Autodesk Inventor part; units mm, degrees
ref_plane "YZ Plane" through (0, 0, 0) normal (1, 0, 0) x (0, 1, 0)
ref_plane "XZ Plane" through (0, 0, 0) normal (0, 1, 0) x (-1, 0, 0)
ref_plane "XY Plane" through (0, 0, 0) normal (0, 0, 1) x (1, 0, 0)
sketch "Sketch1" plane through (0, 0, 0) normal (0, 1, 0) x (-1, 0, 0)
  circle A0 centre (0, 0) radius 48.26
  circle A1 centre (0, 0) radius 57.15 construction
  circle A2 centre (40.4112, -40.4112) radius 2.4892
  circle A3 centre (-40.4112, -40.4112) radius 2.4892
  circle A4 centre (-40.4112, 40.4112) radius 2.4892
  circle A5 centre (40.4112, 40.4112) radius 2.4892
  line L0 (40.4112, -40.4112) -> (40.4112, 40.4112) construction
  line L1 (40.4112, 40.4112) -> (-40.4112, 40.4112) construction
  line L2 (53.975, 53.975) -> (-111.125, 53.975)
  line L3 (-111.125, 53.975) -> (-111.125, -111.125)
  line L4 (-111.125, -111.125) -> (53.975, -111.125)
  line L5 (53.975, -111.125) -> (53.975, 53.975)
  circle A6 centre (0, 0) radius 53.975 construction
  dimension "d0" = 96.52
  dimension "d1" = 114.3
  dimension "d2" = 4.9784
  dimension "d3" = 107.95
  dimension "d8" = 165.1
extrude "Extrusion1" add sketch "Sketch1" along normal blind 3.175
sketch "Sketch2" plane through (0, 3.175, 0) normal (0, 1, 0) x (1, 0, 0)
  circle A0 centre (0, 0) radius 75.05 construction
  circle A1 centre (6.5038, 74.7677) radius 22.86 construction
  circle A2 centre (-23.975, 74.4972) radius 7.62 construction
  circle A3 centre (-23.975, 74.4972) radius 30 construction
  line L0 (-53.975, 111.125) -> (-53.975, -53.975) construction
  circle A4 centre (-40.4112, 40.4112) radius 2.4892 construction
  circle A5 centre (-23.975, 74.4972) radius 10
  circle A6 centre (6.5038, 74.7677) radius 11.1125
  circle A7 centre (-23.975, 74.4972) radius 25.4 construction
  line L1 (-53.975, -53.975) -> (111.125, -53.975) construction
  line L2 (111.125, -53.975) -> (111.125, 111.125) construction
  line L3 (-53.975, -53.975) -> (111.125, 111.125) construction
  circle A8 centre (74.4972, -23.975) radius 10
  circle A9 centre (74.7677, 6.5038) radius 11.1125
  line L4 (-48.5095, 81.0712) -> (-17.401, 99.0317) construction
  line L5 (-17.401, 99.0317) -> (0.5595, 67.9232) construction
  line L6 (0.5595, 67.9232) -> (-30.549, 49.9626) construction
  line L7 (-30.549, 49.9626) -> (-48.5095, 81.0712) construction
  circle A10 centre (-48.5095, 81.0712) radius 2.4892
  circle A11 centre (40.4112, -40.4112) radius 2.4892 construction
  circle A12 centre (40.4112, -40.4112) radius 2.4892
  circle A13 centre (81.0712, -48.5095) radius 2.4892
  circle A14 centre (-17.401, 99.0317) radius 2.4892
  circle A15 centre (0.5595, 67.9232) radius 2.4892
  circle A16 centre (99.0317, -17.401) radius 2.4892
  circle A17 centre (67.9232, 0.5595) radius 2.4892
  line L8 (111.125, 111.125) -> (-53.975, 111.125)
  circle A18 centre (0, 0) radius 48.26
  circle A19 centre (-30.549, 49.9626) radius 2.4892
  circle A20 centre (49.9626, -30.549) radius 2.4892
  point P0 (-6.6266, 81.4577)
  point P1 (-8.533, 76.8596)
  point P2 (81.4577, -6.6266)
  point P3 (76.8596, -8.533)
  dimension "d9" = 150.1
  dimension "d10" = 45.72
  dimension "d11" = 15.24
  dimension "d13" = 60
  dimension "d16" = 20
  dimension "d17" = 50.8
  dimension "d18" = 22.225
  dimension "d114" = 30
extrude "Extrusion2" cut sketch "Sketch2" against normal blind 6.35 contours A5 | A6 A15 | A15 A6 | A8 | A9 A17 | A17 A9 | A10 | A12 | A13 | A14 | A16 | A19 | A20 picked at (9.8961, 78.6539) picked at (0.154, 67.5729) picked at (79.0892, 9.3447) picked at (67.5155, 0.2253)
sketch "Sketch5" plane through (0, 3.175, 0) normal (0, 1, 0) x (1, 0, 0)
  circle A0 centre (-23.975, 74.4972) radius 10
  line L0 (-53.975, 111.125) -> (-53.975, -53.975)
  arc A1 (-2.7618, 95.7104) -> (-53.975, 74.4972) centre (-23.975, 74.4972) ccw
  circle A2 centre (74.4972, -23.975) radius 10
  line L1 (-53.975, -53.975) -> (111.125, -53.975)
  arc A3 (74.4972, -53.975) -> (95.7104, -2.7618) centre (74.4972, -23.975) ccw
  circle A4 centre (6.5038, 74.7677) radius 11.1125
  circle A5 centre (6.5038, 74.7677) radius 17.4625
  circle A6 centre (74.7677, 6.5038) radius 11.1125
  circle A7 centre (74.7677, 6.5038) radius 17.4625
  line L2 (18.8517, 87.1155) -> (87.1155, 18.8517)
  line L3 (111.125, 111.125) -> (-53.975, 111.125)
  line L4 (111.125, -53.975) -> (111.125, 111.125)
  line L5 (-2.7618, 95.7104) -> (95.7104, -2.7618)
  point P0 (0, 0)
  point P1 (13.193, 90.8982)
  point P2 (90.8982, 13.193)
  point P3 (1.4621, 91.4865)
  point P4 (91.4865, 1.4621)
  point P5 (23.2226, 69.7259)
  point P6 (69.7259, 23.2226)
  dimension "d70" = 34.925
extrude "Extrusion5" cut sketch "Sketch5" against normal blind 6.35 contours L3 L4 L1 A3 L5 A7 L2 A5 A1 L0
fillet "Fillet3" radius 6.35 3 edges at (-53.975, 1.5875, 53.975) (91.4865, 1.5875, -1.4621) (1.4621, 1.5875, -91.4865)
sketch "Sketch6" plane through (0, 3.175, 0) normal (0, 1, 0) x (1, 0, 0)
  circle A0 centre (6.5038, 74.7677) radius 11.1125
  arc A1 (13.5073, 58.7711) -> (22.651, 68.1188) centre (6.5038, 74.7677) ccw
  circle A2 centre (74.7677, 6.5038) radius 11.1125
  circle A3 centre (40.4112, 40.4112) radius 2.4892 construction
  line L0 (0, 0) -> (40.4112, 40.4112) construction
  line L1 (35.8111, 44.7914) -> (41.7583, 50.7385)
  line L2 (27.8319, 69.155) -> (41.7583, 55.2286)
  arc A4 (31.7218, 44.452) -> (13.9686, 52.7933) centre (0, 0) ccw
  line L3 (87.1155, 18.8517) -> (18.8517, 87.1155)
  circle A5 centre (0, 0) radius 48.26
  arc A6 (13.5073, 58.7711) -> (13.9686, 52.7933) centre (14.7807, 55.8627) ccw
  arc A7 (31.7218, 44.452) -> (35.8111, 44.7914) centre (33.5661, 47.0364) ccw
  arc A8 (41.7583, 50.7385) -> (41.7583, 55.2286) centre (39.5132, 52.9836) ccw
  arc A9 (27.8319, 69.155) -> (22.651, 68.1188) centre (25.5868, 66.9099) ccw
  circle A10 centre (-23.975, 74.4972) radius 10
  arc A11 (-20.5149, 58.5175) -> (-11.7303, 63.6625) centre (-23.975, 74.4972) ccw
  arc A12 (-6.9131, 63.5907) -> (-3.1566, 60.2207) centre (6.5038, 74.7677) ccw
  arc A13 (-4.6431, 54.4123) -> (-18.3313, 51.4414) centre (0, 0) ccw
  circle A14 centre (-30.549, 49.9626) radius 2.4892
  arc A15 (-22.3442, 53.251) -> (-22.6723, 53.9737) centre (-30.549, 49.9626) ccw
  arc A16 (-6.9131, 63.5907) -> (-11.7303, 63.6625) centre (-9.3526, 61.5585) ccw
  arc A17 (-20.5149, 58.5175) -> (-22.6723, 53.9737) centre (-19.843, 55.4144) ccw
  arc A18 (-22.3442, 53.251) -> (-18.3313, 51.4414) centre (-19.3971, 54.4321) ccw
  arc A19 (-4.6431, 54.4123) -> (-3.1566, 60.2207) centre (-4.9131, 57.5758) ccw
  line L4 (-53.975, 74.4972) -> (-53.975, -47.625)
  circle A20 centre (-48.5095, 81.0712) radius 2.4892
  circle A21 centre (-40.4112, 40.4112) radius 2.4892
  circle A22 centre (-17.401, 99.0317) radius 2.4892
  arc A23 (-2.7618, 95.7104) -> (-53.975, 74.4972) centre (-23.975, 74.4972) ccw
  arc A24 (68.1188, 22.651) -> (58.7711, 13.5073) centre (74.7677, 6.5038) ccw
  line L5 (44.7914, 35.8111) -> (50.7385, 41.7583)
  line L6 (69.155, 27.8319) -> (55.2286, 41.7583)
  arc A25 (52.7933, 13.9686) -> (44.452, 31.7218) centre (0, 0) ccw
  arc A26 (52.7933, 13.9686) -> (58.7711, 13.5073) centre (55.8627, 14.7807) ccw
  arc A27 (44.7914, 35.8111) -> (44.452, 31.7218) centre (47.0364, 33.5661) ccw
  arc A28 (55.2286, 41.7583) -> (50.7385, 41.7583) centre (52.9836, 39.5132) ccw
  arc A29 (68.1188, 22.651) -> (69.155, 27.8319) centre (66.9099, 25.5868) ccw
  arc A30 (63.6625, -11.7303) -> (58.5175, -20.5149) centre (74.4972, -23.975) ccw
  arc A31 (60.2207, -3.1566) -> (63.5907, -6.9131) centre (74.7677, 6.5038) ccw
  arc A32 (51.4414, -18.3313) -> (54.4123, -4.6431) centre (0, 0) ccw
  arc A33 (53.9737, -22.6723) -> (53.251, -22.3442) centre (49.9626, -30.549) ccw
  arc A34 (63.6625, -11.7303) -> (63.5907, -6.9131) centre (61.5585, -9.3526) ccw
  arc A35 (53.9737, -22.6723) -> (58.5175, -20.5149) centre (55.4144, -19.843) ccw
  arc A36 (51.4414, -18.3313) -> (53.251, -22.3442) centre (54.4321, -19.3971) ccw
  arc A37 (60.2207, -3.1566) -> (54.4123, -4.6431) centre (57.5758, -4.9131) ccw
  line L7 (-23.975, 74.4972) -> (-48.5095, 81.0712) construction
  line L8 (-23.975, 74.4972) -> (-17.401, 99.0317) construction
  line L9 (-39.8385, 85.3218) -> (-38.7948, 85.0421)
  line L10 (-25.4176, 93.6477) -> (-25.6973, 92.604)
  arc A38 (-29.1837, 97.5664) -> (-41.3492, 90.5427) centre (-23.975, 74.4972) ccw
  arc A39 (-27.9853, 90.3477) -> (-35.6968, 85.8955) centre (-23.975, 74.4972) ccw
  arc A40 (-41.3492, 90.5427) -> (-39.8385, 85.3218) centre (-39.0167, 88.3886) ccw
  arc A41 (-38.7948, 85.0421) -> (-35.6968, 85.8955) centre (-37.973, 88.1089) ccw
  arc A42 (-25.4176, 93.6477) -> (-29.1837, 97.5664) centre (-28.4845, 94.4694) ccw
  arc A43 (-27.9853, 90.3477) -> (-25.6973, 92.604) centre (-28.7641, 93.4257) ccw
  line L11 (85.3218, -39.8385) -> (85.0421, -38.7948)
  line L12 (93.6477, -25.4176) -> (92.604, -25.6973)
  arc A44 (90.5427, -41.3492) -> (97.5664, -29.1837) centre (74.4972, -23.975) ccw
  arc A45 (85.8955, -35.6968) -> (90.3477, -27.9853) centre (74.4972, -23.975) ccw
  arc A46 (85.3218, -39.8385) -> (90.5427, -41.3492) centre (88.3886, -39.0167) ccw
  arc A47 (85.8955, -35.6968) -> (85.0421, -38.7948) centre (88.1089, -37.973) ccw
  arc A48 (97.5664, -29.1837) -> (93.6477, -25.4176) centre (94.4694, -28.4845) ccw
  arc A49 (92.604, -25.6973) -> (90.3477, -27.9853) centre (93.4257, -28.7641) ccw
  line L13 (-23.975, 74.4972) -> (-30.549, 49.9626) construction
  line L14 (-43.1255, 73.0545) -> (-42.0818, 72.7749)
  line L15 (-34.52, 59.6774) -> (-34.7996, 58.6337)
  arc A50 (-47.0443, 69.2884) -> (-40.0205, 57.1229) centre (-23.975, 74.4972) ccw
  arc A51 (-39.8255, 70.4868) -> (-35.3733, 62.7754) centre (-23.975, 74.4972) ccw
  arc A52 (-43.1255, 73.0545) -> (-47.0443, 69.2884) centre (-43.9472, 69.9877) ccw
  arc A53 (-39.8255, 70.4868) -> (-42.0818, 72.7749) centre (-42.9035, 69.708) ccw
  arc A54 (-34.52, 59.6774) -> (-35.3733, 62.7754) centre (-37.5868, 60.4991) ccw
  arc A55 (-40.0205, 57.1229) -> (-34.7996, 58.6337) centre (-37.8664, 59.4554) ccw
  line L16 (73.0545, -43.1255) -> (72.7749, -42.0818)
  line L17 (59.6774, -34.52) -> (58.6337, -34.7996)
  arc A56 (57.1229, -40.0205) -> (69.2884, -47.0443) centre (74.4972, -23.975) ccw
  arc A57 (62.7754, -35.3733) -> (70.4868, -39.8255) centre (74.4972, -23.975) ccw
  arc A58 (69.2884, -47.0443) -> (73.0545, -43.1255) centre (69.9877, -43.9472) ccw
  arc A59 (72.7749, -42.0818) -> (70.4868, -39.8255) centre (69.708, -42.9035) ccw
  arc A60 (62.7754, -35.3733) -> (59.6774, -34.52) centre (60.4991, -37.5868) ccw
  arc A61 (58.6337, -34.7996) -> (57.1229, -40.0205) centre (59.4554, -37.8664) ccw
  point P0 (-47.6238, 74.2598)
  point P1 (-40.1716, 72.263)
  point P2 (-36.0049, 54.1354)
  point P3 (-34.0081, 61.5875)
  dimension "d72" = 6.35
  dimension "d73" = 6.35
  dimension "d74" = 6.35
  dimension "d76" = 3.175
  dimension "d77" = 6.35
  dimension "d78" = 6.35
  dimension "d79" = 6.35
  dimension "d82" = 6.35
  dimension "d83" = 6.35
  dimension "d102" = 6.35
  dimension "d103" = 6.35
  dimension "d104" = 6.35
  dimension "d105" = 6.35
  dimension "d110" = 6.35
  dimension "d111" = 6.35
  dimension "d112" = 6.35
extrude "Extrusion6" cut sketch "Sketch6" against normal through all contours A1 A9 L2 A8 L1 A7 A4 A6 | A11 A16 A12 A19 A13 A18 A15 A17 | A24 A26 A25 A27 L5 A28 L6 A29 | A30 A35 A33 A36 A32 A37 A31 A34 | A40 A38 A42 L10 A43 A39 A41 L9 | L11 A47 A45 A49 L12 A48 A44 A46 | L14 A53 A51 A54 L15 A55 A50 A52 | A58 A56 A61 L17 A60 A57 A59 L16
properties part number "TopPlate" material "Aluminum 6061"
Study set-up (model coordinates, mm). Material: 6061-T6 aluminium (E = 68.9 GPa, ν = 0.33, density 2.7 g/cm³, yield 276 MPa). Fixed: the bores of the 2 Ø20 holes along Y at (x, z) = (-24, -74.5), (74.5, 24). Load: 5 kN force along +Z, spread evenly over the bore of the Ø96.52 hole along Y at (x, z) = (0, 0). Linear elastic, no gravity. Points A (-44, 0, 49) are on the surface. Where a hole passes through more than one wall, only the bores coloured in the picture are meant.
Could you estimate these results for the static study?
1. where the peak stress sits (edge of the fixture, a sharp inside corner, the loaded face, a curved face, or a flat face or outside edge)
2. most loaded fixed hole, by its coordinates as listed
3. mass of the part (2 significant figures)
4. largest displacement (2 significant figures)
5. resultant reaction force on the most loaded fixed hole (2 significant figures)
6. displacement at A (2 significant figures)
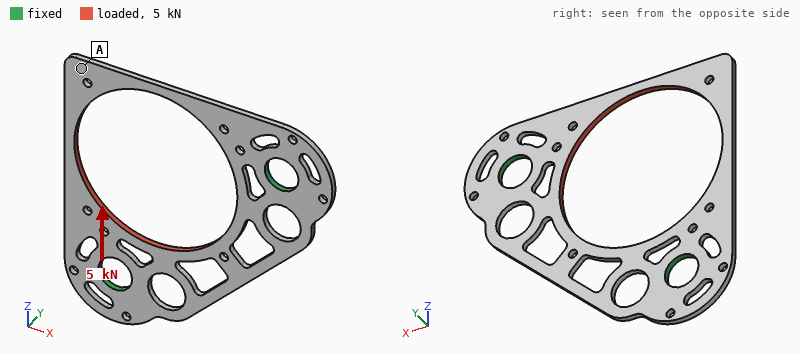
a curved face
(-24, -74.5)
72 g
0.36 mm
2.7 kN
0.17 mm
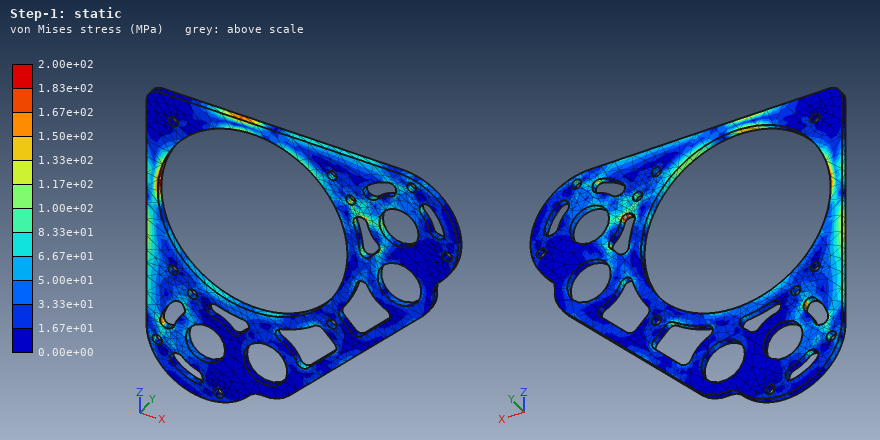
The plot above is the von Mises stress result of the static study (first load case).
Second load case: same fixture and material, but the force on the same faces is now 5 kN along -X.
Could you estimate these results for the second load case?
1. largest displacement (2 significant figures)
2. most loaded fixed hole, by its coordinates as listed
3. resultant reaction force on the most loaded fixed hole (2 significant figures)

0.36 mm
(74.5, 24)
2.7 kN
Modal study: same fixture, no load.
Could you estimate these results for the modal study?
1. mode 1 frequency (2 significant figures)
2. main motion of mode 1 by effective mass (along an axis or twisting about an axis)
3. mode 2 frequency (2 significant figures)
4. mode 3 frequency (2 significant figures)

270 Hz
along Y
890 Hz
910 Hz
